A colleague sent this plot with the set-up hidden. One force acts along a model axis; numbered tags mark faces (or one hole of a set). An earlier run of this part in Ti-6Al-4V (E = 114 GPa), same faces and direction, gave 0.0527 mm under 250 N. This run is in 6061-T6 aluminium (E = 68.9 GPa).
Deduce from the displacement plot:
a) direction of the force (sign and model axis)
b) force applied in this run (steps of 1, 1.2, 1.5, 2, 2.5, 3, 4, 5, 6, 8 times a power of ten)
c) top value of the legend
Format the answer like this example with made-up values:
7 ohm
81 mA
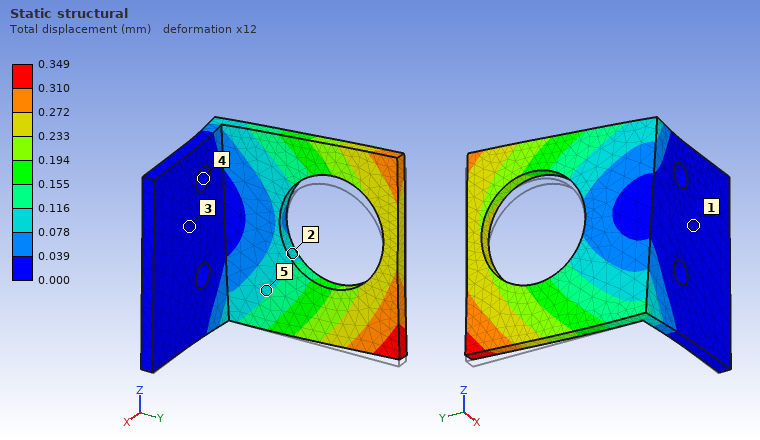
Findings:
+Z
1 kN
0.349 mm
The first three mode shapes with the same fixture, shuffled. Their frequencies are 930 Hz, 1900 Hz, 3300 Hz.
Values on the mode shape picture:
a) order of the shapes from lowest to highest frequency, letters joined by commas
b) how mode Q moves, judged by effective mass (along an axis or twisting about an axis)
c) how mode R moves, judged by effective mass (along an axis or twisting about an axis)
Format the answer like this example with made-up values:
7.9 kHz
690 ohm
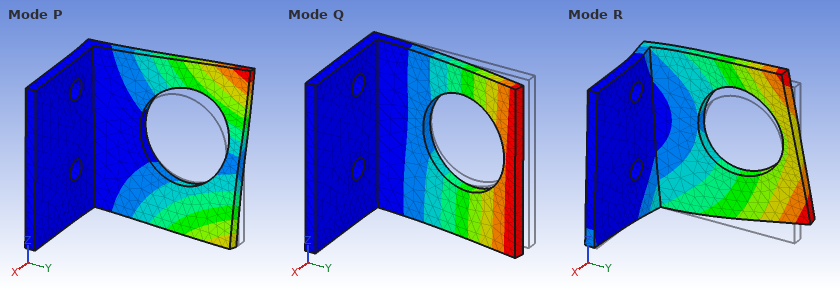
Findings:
Q, P, R
along X
along Z
